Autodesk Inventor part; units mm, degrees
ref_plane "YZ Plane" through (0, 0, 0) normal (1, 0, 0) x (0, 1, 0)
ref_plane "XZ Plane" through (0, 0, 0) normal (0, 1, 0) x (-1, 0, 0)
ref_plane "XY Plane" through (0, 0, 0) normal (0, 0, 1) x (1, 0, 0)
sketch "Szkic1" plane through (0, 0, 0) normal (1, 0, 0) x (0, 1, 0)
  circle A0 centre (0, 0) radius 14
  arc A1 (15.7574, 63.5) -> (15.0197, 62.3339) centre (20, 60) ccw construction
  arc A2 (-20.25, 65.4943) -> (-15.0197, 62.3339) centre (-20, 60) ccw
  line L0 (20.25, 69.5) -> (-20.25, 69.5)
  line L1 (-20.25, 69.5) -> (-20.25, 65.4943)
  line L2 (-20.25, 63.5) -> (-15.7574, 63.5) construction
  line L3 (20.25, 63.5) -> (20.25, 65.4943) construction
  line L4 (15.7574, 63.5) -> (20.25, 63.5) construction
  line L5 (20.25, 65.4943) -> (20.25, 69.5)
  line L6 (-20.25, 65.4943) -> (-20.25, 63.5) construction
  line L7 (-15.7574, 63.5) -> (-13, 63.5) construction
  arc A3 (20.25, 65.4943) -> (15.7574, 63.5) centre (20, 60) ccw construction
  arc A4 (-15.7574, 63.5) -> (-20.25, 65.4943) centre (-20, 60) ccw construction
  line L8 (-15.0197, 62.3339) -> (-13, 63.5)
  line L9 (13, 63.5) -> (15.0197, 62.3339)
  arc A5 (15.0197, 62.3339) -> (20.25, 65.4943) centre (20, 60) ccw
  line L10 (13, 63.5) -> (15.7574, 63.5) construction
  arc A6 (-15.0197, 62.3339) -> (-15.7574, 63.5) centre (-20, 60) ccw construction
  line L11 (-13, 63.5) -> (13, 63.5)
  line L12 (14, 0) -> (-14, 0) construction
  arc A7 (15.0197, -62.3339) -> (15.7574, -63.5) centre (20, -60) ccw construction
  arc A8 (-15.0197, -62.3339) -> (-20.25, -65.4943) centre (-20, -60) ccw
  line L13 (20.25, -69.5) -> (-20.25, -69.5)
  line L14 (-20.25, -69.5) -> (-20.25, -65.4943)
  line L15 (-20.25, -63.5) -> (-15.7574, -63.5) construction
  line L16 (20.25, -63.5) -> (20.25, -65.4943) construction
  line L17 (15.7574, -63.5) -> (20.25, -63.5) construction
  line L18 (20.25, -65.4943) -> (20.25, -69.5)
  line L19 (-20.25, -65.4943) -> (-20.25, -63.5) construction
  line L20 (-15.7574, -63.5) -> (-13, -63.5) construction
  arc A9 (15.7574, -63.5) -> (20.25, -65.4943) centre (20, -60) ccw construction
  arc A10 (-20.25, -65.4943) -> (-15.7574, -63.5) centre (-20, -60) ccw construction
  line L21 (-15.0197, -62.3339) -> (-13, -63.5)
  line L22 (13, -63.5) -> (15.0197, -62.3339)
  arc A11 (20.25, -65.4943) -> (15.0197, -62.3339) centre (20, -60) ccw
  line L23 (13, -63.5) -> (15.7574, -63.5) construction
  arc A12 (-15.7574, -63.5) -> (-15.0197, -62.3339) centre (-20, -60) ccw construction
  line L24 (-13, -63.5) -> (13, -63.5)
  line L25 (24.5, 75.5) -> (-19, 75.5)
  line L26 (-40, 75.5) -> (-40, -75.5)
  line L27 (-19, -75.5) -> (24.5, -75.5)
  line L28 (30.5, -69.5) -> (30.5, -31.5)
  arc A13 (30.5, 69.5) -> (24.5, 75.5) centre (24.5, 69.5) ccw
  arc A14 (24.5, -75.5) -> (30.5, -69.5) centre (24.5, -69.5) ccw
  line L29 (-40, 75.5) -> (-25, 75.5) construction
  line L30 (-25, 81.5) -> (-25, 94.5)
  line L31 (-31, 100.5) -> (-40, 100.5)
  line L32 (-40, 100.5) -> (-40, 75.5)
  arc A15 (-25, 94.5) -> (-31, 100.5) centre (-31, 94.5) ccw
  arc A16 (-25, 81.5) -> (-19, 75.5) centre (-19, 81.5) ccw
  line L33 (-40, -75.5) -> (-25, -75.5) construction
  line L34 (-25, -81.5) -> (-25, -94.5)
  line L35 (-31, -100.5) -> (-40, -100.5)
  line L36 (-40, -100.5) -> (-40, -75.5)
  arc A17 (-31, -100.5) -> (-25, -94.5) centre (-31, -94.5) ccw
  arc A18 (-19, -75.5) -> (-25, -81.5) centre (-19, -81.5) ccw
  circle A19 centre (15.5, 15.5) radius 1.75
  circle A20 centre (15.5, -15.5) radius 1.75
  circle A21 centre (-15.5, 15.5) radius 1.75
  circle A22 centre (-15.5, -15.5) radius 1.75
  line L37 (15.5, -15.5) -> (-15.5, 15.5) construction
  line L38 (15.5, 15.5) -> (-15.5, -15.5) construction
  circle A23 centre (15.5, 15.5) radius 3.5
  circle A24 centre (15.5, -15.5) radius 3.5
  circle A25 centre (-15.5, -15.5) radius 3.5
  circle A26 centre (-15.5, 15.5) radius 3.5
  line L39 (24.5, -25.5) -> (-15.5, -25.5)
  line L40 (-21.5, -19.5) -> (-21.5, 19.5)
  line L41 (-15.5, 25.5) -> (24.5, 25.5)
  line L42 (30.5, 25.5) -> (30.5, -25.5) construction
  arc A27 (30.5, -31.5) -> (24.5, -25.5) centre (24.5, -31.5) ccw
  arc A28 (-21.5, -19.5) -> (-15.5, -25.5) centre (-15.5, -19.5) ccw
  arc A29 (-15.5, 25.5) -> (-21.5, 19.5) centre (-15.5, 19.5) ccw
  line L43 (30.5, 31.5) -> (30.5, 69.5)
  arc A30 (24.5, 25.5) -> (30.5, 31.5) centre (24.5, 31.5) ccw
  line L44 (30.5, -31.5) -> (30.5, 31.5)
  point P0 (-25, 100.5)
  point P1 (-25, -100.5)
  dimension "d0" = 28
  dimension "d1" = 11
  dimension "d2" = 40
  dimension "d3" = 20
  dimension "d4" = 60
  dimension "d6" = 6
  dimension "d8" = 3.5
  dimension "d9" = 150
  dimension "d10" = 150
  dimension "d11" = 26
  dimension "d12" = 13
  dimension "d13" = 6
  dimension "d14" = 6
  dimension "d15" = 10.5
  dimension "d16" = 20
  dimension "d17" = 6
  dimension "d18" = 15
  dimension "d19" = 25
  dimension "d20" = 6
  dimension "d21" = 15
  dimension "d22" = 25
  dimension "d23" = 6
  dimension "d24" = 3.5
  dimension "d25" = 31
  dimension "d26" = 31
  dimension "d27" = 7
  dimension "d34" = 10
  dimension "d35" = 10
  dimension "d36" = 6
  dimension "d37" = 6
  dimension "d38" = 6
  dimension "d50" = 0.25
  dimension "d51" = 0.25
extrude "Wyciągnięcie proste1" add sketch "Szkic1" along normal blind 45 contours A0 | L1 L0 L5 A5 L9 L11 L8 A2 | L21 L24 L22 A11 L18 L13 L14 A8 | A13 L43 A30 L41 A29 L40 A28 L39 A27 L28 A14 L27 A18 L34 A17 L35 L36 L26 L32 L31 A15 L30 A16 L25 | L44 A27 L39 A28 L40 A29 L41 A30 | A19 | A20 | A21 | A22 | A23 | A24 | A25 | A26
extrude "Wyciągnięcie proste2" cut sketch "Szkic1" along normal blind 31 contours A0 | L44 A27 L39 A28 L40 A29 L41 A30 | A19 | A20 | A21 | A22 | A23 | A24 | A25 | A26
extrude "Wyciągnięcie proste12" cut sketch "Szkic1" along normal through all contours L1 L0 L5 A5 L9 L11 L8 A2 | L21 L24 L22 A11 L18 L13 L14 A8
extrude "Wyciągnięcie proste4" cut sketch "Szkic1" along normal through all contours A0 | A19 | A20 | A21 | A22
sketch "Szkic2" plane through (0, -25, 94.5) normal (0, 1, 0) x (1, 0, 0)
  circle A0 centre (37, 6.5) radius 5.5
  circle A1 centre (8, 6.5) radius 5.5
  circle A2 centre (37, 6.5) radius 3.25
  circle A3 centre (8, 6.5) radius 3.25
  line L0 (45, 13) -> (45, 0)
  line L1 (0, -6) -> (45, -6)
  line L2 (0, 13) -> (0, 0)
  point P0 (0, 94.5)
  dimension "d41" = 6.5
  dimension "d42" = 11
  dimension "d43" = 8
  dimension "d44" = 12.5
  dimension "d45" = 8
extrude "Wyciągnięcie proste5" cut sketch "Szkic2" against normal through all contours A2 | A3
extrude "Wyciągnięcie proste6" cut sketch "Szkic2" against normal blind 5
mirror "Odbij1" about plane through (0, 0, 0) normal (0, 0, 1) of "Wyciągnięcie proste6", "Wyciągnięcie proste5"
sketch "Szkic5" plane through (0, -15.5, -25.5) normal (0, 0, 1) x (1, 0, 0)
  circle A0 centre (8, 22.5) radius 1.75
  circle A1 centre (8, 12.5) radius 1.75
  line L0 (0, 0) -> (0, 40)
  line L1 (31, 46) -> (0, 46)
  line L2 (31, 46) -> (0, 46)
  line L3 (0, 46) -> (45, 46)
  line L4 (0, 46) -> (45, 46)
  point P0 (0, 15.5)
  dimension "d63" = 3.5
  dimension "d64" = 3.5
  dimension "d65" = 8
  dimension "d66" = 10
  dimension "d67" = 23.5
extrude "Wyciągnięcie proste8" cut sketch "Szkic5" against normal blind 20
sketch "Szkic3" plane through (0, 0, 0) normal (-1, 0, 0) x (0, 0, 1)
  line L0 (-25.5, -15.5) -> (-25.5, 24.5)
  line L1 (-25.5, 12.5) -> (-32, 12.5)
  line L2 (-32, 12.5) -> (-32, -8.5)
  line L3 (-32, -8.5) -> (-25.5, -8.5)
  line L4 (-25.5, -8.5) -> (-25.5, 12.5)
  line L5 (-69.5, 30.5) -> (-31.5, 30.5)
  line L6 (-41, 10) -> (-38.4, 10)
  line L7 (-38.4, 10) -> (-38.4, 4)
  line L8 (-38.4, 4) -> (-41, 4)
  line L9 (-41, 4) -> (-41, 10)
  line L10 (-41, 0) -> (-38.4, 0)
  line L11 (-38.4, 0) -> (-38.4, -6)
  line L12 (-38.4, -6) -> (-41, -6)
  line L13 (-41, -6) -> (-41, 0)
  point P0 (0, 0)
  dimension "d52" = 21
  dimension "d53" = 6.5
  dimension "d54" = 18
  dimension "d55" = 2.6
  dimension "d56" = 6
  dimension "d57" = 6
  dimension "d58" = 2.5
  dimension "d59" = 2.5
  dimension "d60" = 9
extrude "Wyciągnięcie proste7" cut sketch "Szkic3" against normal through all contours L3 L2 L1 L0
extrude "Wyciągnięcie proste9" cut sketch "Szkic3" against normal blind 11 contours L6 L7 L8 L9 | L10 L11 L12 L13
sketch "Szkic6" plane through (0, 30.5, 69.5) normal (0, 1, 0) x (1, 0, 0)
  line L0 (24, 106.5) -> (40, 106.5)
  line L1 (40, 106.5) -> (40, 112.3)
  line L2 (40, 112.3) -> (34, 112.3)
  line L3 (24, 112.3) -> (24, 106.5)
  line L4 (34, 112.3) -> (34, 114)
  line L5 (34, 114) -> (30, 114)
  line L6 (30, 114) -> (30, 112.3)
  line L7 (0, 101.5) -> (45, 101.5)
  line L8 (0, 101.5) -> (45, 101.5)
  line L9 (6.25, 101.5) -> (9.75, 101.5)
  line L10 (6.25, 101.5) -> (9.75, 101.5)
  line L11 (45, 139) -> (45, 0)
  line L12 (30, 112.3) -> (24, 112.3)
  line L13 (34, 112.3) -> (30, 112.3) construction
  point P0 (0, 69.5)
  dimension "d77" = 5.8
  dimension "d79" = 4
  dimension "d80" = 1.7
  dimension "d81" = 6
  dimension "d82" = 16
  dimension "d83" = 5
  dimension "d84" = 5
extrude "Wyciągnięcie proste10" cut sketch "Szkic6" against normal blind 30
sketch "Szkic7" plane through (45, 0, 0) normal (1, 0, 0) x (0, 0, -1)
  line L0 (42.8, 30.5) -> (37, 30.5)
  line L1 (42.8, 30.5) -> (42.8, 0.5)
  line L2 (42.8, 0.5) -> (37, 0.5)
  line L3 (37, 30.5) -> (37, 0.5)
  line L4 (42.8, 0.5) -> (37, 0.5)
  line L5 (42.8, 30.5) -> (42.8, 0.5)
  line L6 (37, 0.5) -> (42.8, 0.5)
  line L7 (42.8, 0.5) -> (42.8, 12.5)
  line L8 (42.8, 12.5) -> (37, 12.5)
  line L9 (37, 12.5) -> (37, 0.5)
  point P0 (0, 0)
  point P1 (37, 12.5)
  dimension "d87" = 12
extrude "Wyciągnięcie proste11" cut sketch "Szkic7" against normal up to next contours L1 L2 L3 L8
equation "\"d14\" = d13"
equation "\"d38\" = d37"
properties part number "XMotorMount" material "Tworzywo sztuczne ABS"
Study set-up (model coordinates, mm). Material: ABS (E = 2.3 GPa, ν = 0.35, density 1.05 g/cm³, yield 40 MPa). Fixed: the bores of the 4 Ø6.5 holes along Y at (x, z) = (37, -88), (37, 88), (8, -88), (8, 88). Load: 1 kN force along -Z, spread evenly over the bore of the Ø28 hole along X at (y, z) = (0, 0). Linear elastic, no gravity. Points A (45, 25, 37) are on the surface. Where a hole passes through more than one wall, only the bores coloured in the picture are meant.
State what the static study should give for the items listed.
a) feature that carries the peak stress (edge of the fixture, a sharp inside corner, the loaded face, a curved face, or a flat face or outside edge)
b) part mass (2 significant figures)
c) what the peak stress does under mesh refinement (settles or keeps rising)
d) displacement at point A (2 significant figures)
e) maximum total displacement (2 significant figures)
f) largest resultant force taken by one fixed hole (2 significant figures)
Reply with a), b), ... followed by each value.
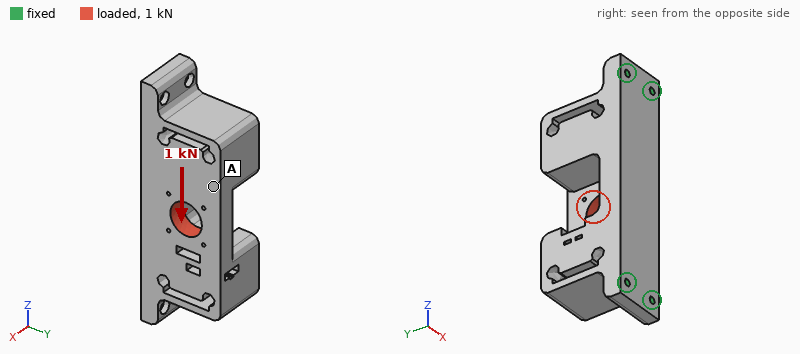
a) edge of the fixture
b) 390 g
c) keeps rising
d) 74 µm
e) 80 µm
f) 310 N
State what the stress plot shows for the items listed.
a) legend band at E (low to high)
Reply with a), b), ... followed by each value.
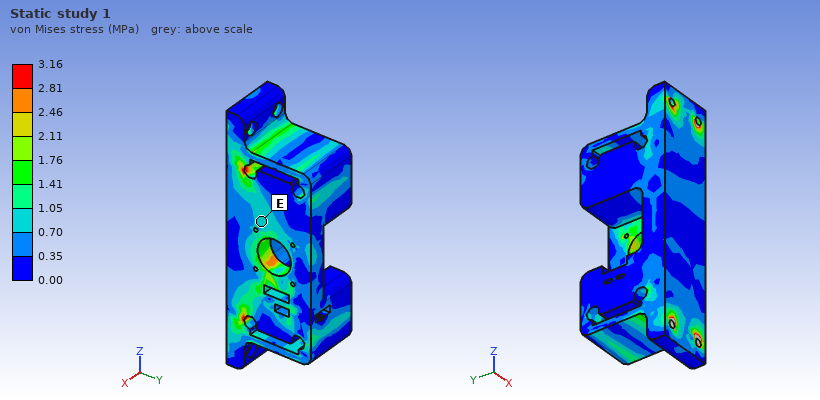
a) 0.70 to 1.05 MPa
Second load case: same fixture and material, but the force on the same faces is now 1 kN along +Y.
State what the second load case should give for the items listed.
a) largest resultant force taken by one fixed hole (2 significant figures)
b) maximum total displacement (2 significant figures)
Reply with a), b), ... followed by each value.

a) 610 N
b) 0.38 mm
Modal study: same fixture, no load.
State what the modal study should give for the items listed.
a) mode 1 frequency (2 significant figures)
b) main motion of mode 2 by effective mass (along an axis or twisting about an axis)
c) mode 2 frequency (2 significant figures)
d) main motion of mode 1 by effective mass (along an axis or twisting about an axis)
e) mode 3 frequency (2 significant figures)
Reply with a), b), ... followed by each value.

a) 540 Hz
b) along Y
c) 740 Hz
d) along X
e) 1000 Hz
